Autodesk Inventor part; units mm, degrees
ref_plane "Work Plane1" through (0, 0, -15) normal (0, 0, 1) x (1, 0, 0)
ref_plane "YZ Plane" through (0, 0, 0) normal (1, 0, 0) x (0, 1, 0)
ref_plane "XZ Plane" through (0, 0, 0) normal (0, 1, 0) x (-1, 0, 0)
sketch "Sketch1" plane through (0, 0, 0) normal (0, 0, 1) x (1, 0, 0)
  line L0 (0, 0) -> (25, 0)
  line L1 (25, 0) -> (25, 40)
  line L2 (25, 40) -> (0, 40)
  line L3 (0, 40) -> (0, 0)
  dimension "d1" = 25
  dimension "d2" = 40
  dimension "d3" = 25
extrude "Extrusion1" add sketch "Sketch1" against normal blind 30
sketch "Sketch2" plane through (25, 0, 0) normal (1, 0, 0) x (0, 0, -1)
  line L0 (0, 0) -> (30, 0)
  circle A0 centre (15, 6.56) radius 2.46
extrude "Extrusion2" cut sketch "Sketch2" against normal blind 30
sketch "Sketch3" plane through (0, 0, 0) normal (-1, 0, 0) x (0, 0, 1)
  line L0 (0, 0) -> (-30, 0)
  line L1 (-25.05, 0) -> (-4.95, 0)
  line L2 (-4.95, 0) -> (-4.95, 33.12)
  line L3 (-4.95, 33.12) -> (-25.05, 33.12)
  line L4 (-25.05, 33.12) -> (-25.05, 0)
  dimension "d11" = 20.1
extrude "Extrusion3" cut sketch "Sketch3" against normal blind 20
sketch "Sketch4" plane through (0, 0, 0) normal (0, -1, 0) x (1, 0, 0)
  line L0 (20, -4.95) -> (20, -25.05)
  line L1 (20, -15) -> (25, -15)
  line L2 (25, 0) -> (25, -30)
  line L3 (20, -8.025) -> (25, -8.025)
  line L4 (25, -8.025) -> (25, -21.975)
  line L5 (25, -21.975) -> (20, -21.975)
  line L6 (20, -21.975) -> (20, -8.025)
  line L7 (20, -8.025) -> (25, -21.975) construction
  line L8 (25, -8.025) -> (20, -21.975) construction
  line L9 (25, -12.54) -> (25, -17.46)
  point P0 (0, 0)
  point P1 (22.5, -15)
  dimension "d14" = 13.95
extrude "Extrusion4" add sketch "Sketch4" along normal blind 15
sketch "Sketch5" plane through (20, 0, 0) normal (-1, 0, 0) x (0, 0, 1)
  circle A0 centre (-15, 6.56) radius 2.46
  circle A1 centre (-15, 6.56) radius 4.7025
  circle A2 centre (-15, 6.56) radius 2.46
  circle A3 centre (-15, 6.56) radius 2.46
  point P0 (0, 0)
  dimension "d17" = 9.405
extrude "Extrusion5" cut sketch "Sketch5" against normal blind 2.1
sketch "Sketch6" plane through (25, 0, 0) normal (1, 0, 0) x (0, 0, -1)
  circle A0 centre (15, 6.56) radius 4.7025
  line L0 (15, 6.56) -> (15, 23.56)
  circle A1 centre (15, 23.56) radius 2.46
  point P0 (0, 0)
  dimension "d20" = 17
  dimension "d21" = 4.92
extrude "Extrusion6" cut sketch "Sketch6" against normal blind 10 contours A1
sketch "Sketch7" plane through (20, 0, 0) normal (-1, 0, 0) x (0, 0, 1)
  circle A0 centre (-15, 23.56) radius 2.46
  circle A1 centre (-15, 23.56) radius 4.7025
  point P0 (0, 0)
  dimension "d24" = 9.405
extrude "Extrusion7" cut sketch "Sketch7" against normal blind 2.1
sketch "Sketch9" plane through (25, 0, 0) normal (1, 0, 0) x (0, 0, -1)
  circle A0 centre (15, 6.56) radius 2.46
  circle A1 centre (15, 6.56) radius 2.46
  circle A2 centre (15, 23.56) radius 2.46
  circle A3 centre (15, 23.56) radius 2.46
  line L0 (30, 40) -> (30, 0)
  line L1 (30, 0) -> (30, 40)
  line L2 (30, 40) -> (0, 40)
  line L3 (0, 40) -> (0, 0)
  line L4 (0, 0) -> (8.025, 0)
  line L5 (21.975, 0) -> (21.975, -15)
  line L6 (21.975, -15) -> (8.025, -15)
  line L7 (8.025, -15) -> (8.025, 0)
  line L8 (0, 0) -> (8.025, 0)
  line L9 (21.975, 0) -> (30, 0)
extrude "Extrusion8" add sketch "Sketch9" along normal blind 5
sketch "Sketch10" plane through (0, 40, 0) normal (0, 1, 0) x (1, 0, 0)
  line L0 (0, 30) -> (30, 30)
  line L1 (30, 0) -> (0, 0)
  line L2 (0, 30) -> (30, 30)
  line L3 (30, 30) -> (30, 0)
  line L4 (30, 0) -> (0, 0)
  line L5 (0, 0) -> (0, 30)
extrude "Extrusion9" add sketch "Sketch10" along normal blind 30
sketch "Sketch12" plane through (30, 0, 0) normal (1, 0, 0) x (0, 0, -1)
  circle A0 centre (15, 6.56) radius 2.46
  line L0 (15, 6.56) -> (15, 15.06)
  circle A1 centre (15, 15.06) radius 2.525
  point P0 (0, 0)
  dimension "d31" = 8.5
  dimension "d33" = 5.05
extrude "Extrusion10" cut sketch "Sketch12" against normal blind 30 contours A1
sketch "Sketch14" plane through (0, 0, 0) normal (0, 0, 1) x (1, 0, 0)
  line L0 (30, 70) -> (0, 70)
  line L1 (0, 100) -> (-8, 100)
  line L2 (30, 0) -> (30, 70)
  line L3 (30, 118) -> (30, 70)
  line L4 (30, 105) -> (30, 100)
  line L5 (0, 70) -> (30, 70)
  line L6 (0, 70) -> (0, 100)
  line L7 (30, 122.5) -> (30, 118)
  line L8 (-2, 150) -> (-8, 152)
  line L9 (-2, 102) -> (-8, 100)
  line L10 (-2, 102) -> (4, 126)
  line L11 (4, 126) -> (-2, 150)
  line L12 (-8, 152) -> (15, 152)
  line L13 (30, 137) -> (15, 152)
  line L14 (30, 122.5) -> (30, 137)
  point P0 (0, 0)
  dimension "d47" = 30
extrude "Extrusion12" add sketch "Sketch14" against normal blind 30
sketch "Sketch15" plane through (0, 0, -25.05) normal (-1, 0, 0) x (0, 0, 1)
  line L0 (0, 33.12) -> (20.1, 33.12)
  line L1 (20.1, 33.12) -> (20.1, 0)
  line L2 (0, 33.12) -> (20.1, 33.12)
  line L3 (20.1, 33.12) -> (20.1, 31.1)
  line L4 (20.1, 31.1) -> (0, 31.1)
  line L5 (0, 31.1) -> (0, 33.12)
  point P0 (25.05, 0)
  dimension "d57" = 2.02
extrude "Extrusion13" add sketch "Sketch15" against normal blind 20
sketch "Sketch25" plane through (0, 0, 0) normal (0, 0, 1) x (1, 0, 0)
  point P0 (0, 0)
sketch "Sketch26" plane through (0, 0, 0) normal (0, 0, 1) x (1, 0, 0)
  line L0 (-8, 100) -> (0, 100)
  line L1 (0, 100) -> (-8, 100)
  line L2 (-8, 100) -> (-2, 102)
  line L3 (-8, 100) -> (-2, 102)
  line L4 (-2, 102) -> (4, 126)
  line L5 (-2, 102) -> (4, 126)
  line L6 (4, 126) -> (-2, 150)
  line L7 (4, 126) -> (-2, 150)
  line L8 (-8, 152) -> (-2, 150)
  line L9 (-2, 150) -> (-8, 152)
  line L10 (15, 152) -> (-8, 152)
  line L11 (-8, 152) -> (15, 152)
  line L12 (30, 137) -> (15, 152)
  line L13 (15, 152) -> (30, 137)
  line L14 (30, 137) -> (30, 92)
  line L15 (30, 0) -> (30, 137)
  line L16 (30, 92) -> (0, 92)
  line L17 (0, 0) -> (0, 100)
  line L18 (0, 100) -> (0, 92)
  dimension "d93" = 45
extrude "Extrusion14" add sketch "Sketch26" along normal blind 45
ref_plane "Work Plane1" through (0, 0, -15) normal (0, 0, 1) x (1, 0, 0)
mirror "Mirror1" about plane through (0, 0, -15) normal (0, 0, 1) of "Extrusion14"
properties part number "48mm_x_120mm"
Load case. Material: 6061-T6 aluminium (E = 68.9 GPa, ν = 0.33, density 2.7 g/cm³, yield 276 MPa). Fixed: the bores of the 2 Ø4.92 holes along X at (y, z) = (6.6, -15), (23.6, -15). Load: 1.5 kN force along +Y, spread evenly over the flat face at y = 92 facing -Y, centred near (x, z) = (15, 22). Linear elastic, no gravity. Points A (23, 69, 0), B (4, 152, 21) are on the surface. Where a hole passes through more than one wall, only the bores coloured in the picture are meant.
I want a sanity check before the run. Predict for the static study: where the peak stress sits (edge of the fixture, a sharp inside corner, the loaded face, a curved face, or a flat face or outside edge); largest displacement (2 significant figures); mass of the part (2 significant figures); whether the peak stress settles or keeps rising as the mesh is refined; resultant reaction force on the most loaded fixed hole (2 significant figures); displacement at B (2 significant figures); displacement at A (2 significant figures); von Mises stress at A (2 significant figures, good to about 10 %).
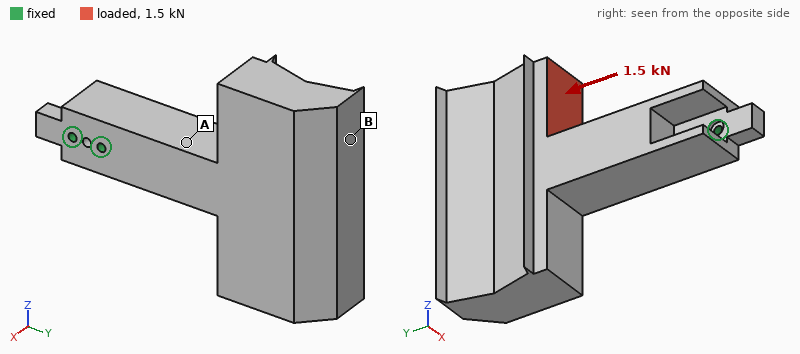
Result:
edge of the fixture
0.23 mm
730 g
keeps rising
2.7 kN
0.20 mm
0.057 mm
14 MPa
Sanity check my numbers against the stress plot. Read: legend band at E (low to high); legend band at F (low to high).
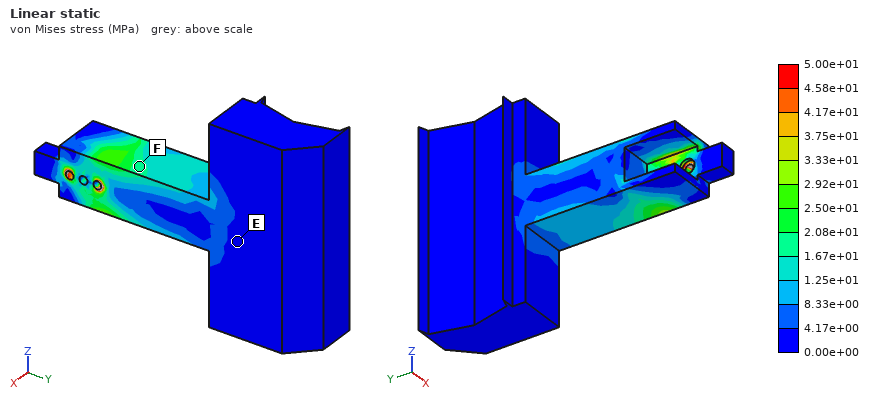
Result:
0.00e+00 to 4.17e+00 MPa
1.67e+01 to 2.08e+01 MPa
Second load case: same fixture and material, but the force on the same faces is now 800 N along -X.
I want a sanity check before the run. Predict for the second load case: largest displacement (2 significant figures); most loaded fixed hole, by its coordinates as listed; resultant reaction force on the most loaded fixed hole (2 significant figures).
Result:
0.32 mm
(23.6, -15)
2.9 kN
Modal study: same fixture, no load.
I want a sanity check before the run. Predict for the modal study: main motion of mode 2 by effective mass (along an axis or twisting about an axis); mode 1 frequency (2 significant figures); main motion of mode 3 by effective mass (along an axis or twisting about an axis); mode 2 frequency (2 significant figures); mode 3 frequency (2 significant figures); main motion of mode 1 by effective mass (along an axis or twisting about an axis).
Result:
along Z
400 Hz
twisting about Y
440 Hz
720 Hz
along X
